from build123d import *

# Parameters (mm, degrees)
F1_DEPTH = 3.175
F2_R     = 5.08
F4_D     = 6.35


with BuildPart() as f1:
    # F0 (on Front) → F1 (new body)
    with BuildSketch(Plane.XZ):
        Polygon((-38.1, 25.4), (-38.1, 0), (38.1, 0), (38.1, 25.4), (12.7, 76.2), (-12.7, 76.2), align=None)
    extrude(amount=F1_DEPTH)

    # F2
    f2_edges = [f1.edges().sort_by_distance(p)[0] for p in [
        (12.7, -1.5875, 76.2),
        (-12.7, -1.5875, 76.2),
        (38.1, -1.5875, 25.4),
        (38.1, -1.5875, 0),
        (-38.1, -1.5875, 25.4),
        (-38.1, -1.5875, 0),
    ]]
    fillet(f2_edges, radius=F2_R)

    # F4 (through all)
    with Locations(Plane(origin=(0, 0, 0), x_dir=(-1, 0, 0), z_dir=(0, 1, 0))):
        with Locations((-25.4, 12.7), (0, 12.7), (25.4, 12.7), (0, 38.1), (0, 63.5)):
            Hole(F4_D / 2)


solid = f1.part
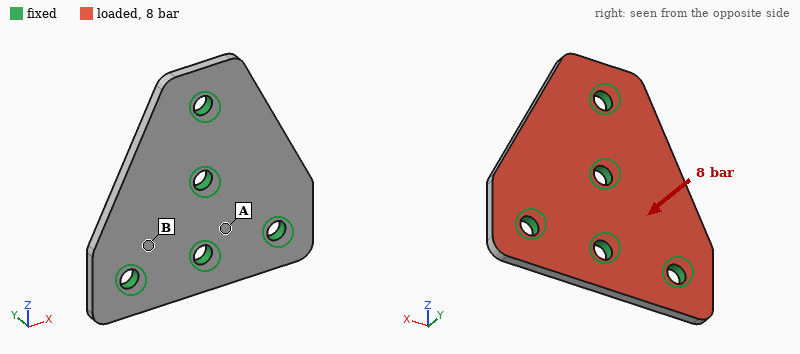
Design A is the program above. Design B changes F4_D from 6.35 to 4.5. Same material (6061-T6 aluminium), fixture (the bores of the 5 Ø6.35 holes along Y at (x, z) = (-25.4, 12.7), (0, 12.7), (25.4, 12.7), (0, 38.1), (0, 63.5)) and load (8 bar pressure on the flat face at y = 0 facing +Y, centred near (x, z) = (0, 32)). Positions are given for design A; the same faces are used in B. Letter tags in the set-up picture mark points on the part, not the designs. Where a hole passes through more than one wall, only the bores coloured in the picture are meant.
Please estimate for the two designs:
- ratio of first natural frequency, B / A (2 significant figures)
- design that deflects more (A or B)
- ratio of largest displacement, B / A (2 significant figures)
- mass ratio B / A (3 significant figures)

0.89
B
1.1
1.02
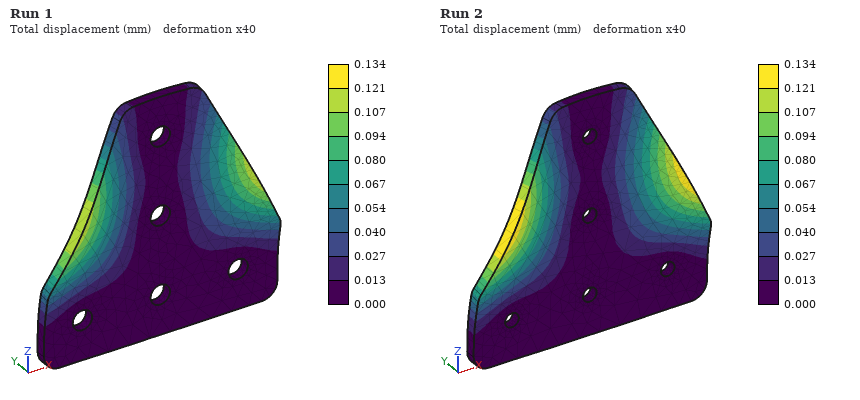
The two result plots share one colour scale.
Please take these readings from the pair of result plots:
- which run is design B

Run 2
